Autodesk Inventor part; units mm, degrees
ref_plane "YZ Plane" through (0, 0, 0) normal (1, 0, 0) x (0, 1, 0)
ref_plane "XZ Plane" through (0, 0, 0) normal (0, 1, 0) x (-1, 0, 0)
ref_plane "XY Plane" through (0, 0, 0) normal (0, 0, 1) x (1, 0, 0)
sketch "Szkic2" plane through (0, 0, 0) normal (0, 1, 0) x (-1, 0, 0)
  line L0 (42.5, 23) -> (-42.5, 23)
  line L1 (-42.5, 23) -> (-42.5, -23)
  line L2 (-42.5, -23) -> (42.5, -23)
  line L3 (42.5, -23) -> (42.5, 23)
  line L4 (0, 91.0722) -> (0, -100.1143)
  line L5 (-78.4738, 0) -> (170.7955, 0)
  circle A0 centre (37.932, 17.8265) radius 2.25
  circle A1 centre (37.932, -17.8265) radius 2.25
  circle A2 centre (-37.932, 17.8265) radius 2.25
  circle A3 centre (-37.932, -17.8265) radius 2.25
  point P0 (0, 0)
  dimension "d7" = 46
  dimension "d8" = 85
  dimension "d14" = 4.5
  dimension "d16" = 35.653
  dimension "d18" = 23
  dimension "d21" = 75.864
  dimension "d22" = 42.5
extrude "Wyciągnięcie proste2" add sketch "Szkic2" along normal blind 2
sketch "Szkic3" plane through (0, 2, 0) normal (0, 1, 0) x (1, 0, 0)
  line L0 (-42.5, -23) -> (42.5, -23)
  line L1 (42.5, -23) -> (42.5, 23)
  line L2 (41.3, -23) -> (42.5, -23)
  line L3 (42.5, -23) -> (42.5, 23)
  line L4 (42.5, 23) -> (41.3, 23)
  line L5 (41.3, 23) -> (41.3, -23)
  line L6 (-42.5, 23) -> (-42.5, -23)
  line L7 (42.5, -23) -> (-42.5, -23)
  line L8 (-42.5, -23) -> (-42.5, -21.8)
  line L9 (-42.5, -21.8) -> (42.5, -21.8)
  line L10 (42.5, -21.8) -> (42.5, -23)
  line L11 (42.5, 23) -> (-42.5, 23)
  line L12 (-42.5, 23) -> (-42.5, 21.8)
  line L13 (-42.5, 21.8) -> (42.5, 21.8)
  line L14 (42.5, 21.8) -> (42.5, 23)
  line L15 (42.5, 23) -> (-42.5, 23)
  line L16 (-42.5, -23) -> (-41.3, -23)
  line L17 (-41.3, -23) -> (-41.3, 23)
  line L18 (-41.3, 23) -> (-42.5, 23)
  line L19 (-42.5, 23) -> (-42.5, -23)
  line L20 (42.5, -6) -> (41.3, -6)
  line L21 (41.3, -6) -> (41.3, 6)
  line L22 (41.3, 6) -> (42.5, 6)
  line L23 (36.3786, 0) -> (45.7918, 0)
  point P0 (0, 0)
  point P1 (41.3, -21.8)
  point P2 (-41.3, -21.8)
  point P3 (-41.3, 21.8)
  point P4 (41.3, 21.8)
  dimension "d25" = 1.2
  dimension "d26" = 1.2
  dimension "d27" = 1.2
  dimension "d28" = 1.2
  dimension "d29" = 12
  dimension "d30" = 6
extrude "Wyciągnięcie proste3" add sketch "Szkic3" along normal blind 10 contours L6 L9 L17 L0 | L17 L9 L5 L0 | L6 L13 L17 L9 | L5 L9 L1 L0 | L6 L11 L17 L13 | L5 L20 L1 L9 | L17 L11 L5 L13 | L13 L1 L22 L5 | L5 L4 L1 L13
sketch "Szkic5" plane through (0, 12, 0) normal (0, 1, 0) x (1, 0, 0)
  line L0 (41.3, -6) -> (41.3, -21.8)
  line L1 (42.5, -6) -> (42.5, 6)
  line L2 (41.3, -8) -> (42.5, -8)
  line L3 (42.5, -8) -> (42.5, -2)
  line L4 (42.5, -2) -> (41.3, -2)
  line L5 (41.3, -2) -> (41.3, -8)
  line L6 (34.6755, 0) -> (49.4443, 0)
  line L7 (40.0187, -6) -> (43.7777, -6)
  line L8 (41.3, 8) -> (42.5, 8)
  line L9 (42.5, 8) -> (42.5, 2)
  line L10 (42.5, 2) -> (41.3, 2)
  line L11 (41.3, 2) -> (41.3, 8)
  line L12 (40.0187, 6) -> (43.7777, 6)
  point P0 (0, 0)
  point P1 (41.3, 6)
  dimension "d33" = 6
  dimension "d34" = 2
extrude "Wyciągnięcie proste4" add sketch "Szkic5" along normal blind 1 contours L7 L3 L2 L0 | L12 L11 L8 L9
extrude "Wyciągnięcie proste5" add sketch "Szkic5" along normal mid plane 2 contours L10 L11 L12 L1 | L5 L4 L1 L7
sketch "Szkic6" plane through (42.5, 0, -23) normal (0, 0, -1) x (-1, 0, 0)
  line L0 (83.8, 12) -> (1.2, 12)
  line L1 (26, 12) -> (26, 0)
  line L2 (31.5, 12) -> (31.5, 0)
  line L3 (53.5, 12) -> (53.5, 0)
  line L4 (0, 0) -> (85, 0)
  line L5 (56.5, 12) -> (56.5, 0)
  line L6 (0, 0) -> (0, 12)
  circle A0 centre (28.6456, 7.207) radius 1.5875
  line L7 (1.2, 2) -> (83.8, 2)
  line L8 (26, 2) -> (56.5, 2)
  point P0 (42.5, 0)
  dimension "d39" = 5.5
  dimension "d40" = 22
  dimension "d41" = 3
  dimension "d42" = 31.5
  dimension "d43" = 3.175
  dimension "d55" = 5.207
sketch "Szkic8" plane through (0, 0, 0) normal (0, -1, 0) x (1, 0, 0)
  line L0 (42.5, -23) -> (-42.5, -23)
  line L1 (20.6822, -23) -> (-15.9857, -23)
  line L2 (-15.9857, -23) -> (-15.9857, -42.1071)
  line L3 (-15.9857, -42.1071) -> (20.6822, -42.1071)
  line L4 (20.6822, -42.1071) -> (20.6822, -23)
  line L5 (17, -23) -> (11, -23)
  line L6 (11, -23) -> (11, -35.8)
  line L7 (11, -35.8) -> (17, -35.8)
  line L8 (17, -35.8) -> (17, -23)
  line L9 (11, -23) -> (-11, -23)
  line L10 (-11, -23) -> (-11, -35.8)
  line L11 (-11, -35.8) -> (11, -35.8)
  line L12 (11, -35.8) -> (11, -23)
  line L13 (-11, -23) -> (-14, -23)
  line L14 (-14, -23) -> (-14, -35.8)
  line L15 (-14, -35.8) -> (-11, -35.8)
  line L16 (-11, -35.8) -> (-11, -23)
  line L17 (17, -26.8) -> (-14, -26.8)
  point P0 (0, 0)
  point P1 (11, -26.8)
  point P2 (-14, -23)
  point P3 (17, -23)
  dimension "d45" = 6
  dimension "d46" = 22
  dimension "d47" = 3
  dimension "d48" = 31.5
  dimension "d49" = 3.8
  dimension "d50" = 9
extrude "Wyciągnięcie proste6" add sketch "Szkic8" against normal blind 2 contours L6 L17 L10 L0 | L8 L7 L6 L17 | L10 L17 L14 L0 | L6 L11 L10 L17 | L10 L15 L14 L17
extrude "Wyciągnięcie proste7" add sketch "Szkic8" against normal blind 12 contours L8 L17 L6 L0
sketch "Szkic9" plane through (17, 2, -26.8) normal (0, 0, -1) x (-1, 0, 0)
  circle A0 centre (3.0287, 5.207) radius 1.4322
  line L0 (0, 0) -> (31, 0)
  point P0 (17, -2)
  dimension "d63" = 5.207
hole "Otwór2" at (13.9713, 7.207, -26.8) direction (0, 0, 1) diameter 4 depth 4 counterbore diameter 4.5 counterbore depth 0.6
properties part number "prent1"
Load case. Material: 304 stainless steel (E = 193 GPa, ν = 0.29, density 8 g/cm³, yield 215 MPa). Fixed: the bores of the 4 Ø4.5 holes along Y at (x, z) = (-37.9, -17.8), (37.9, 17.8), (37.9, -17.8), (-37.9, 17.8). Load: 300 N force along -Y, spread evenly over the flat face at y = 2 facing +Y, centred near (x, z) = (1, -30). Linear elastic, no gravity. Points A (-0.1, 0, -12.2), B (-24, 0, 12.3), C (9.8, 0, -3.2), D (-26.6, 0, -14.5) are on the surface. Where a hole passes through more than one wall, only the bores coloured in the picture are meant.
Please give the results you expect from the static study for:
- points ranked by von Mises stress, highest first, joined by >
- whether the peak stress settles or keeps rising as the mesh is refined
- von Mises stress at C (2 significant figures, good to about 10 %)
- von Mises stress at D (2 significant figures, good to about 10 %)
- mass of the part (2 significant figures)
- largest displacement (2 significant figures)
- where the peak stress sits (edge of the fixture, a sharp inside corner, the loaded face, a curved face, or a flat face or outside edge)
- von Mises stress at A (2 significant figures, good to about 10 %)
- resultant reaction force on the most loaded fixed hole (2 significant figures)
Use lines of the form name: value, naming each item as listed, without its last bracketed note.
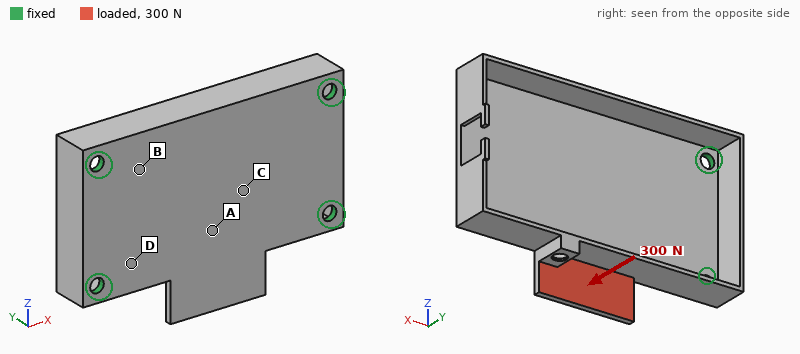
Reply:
points ranked by von Mises stress, highest first, joined by >: A > D > C > B
whether the peak stress settles or keeps rising as the mesh is refined: keeps rising
von Mises stress at C: 20 MPa
von Mises stress at D: 30 MPa
mass of the part: 93 g
largest displacement: 0.11 mm
where the peak stress sits: edge of the fixture
von Mises stress at A: 40 MPa
resultant reaction force on the most loaded fixed hole: 310 N
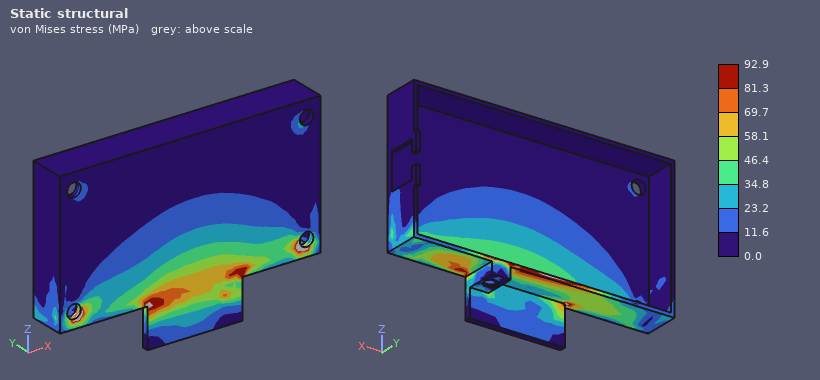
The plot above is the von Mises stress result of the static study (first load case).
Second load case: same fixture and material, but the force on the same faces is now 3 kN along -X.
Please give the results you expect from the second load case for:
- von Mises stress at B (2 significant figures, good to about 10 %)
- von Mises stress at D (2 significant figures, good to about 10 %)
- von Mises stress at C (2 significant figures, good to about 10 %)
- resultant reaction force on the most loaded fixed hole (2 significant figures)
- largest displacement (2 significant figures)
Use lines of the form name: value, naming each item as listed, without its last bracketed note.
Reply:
von Mises stress at B: 14 MPa
von Mises stress at D: 36 MPa
von Mises stress at C: 11 MPa
resultant reaction force on the most loaded fixed hole: 1.2 kN
largest displacement: 33 µm
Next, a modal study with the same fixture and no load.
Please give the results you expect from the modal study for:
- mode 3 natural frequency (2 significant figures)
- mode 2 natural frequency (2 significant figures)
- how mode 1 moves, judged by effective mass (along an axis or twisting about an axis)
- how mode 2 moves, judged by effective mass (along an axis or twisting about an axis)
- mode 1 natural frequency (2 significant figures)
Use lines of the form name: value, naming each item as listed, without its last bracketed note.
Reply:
mode 3 natural frequency: 5700 Hz
mode 2 natural frequency: 3500 Hz
how mode 1 moves, judged by effective mass: along Y
how mode 2 moves, judged by effective mass: along Y
mode 1 natural frequency: 2900 Hz
